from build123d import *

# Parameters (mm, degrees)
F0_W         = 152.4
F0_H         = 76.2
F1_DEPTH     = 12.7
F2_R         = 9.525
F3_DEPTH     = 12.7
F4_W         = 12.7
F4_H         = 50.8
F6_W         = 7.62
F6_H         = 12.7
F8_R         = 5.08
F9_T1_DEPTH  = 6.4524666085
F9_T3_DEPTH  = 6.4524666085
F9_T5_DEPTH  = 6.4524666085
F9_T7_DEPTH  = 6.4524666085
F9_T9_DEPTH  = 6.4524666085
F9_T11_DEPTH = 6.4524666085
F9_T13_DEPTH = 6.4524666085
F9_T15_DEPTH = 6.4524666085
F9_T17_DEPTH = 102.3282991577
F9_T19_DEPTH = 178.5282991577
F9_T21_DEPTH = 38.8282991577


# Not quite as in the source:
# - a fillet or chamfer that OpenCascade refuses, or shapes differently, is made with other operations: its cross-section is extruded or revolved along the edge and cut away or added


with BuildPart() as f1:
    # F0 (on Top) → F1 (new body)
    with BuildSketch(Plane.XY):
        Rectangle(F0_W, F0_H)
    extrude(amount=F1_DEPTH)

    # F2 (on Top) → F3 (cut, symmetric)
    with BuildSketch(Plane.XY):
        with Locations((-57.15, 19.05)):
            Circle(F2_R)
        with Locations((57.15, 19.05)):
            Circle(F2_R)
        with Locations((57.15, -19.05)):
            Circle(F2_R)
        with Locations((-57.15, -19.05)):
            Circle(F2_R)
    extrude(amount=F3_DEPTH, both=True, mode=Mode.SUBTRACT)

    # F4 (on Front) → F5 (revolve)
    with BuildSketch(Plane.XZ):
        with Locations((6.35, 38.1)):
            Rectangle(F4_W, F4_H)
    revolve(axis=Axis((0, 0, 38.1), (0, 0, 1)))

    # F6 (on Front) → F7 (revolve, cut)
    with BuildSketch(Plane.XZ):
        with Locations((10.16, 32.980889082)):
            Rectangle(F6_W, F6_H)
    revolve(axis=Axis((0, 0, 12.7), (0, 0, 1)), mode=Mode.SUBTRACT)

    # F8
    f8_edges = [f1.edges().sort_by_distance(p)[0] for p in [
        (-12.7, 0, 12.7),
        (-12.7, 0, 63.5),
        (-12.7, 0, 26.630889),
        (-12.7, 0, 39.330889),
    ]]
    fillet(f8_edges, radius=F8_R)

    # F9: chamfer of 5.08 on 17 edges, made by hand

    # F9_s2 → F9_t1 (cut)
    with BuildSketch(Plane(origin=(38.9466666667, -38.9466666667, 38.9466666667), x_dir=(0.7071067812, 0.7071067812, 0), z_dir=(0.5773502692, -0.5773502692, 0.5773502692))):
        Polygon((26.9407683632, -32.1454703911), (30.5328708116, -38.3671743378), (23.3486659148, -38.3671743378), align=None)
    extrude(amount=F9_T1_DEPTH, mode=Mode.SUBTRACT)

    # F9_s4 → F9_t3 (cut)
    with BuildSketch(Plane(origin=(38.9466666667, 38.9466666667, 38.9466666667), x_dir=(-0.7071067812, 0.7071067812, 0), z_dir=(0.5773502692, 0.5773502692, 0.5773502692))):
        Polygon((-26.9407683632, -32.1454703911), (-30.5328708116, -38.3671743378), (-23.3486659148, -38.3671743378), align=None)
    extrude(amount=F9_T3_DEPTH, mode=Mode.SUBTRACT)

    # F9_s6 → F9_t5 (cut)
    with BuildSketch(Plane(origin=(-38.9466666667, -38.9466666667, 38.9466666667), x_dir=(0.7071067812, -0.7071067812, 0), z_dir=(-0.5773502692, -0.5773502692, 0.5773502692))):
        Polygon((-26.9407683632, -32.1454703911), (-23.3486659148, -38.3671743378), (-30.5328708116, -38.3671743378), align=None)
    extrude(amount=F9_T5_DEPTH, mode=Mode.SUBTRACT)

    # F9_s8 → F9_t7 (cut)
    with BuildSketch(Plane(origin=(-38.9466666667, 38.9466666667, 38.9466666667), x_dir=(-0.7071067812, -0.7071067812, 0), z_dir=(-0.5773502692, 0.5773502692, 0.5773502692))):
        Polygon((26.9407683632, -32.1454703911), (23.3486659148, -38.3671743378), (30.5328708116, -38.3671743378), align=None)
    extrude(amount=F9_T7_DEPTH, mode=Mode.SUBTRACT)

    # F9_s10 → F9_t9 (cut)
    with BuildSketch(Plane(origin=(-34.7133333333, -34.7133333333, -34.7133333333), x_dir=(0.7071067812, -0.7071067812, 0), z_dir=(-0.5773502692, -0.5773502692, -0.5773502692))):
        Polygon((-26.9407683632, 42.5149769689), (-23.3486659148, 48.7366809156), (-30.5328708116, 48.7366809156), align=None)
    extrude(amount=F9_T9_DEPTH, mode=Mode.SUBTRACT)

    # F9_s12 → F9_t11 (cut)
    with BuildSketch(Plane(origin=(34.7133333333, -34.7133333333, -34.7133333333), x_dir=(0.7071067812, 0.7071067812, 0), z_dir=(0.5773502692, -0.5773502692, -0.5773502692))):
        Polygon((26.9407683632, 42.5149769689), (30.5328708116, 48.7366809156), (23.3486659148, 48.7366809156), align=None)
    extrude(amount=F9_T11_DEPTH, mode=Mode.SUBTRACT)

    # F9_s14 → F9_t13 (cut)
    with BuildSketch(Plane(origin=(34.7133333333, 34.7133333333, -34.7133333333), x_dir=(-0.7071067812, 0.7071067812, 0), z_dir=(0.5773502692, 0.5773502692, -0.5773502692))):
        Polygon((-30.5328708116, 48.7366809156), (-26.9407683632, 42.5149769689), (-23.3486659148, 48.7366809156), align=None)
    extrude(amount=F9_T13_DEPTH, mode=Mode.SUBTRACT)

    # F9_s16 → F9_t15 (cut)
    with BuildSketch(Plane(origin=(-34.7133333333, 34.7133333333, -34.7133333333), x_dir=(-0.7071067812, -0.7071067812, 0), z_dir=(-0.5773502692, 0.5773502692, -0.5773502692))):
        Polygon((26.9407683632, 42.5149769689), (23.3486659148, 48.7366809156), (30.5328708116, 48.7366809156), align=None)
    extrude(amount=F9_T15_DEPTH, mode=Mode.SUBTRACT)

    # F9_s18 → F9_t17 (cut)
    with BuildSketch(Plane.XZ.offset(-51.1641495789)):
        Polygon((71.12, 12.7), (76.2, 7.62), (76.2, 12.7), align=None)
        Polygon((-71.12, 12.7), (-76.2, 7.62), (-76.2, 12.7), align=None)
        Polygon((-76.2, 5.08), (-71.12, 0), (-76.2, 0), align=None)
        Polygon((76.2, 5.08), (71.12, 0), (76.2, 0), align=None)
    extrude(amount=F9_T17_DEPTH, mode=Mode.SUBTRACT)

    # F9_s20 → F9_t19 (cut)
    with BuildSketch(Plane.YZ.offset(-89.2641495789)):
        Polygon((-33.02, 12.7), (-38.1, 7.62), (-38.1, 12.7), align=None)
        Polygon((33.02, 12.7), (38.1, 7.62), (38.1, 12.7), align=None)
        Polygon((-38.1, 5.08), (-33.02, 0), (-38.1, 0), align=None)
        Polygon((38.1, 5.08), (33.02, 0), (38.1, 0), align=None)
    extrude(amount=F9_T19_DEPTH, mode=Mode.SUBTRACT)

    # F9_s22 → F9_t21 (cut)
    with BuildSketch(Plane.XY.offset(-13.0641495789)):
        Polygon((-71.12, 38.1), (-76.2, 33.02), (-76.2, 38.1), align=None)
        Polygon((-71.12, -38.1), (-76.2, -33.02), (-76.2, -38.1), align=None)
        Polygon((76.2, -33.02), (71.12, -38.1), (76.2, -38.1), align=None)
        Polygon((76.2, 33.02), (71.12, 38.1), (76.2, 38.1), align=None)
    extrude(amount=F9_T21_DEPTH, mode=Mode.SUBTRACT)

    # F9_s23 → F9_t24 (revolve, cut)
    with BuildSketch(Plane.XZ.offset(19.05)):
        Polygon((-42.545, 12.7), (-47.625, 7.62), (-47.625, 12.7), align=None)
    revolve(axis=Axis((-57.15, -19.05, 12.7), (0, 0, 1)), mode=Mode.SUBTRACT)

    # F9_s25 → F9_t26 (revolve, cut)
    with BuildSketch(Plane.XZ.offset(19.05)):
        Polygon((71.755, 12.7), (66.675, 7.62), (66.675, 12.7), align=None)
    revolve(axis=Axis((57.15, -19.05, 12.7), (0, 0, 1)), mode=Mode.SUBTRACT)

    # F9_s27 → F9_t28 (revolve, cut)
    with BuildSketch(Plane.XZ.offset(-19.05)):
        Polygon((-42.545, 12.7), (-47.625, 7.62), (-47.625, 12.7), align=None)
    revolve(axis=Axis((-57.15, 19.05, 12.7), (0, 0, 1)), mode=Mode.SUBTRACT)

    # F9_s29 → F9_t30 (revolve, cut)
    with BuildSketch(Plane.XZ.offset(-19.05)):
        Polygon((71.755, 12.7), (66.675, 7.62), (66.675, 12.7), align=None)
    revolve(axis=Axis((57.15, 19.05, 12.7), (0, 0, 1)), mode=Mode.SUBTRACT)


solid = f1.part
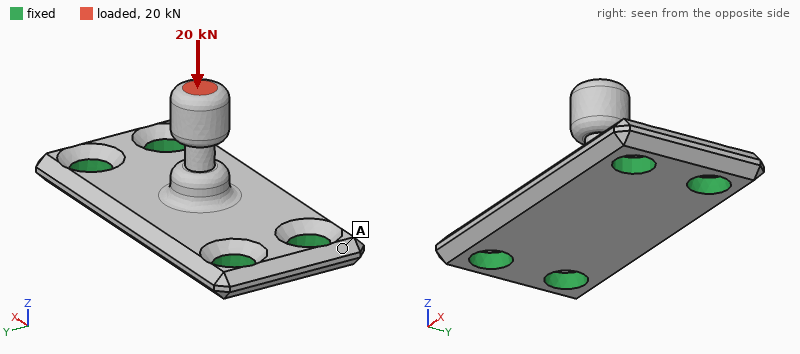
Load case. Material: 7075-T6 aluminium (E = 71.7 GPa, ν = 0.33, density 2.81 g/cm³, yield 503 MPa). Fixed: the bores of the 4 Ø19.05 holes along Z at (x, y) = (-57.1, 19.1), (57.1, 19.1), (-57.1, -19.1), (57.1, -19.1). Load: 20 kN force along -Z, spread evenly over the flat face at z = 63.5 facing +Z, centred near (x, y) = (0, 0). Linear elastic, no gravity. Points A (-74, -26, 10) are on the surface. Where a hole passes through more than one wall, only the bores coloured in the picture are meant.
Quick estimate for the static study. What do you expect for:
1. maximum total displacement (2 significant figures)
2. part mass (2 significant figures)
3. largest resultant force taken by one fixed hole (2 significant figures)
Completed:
0.21 mm
390 g
6.4 kN
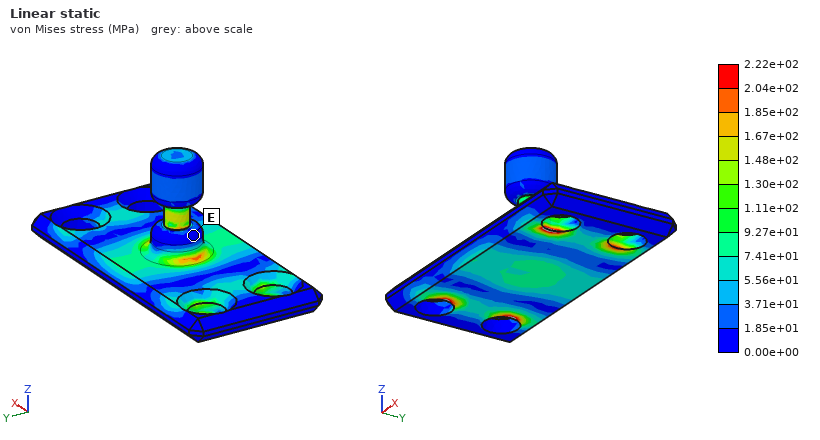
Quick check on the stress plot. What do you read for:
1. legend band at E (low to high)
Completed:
0.00e+00 to 1.85e+01 MPa
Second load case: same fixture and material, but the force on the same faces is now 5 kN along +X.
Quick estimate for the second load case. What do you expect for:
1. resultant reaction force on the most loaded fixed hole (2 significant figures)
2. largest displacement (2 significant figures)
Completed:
2.3 kN
1.2 mm
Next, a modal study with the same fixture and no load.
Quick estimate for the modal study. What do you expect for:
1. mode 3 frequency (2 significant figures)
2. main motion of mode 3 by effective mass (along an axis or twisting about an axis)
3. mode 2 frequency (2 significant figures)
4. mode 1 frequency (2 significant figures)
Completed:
4500 Hz
along Z
2600 Hz
2500 Hz
